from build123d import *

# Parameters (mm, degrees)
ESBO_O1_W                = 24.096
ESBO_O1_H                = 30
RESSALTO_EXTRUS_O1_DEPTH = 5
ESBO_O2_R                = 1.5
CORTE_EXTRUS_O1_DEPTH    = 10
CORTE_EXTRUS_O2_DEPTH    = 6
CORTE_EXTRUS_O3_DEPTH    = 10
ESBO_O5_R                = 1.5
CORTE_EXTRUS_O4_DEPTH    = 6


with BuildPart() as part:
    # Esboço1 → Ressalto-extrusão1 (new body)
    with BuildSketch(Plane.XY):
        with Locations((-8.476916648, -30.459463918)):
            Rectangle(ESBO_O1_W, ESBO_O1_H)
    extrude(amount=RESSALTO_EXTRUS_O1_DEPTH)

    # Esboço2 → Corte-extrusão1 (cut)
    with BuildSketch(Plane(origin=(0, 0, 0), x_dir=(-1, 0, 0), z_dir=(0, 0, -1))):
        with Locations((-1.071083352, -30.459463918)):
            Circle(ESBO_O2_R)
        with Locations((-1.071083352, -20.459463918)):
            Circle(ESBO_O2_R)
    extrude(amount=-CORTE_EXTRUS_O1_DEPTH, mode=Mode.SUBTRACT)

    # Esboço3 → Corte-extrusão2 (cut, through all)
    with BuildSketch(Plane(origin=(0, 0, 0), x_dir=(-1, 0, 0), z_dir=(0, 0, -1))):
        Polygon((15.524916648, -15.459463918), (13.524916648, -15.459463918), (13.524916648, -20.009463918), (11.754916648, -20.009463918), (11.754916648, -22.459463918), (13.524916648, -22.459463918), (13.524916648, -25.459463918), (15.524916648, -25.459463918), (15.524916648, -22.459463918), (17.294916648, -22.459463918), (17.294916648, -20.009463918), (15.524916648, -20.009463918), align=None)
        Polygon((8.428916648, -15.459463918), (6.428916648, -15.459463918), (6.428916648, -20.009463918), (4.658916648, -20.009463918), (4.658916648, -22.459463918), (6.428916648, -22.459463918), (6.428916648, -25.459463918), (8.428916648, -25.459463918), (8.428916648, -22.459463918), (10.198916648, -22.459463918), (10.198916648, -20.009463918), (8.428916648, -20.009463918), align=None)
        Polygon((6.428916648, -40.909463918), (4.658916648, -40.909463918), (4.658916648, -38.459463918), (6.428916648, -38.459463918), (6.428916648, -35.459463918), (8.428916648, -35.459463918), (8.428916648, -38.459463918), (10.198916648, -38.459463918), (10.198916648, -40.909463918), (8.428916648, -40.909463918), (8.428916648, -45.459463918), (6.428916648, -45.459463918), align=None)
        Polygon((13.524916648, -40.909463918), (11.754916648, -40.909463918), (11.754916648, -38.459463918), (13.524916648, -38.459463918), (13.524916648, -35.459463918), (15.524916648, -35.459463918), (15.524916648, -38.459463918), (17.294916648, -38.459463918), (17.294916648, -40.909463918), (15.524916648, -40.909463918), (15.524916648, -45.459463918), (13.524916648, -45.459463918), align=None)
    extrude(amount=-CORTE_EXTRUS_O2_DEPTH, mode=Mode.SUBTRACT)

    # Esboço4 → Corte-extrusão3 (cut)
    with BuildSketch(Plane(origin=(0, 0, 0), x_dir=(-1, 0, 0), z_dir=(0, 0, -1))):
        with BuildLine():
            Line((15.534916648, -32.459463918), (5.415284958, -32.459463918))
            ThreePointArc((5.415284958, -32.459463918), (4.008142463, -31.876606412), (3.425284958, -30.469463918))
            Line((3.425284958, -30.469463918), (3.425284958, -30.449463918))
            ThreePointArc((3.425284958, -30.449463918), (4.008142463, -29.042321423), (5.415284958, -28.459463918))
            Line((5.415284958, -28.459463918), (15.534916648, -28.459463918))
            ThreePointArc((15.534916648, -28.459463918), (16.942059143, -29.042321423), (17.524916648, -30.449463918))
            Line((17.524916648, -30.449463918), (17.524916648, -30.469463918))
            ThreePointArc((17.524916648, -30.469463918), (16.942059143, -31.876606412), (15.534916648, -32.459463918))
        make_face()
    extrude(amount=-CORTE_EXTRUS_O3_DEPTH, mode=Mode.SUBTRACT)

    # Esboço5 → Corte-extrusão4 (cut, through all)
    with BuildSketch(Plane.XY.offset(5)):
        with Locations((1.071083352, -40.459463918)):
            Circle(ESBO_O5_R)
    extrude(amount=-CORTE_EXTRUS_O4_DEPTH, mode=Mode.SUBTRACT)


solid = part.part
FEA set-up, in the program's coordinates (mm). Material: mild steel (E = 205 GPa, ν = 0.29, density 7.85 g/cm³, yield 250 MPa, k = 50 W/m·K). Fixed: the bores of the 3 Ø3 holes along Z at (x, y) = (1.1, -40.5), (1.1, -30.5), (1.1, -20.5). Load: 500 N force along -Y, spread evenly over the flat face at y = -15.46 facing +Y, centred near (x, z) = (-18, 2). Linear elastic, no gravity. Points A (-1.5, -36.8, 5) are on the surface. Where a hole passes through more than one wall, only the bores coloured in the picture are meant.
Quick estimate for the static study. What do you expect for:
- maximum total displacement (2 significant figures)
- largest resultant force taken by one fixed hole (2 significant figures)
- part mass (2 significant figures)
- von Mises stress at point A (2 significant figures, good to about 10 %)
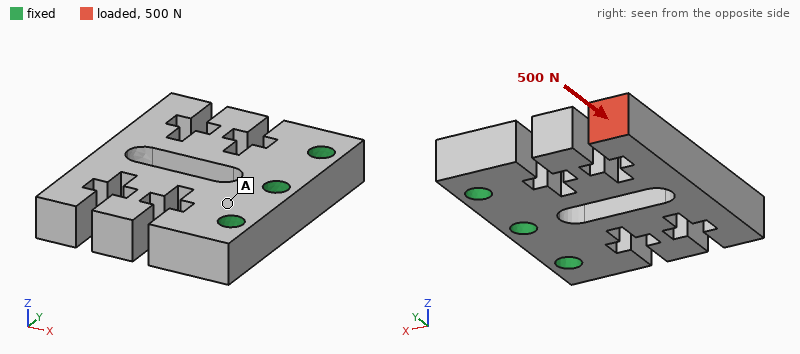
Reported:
33 µm
530 N
21 g
19 MPa
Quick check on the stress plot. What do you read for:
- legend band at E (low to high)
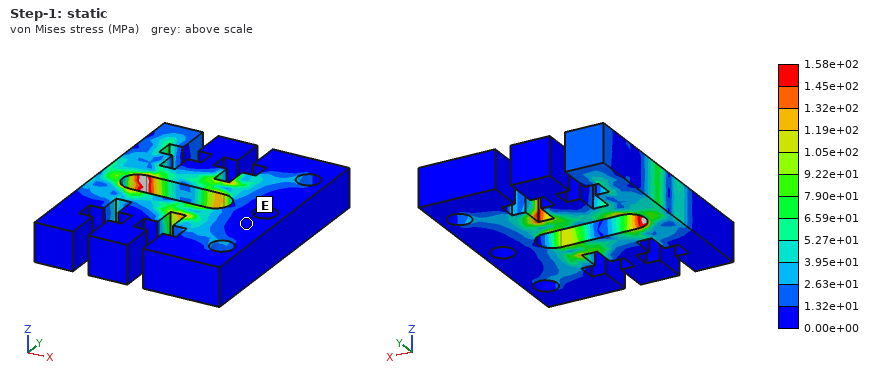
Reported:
0.00e+00 to 1.32e+01 MPa
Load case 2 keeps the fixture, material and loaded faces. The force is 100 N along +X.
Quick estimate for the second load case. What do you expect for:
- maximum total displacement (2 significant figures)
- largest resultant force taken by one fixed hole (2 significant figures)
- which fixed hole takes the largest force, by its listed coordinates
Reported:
18 µm
140 N
(1.1, -30.5)
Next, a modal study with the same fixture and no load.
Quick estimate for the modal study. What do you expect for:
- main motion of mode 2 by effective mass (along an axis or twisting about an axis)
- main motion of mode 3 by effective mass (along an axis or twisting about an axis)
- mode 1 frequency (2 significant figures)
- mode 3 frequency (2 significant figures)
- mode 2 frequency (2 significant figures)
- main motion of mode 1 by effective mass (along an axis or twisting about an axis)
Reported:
twisting about X
along Y
5800 Hz
7300 Hz
6200 Hz
along Z
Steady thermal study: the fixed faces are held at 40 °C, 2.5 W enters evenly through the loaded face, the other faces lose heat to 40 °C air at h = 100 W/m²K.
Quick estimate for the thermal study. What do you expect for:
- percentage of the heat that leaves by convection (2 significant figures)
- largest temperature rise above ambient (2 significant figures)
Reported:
54 %
38 K
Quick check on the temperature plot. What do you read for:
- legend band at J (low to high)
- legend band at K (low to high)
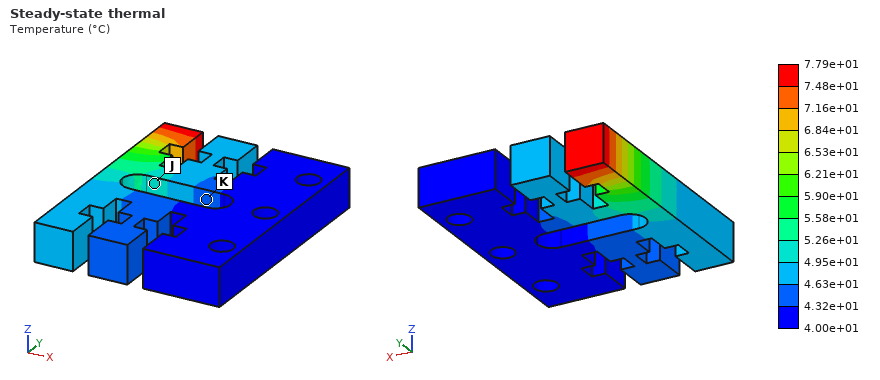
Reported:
4.95e+01 to 5.26e+01 °C
4.32e+01 to 4.63e+01 °C
